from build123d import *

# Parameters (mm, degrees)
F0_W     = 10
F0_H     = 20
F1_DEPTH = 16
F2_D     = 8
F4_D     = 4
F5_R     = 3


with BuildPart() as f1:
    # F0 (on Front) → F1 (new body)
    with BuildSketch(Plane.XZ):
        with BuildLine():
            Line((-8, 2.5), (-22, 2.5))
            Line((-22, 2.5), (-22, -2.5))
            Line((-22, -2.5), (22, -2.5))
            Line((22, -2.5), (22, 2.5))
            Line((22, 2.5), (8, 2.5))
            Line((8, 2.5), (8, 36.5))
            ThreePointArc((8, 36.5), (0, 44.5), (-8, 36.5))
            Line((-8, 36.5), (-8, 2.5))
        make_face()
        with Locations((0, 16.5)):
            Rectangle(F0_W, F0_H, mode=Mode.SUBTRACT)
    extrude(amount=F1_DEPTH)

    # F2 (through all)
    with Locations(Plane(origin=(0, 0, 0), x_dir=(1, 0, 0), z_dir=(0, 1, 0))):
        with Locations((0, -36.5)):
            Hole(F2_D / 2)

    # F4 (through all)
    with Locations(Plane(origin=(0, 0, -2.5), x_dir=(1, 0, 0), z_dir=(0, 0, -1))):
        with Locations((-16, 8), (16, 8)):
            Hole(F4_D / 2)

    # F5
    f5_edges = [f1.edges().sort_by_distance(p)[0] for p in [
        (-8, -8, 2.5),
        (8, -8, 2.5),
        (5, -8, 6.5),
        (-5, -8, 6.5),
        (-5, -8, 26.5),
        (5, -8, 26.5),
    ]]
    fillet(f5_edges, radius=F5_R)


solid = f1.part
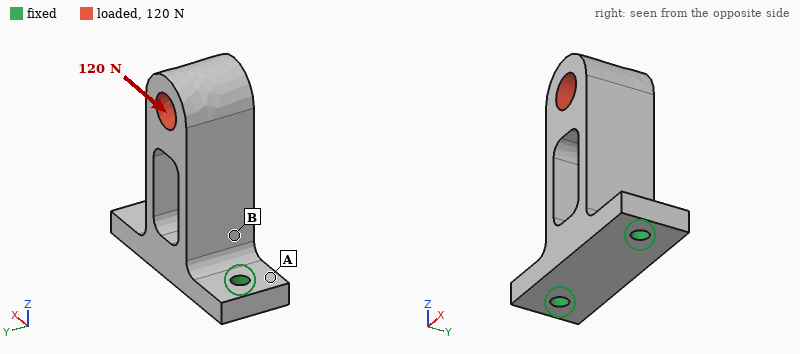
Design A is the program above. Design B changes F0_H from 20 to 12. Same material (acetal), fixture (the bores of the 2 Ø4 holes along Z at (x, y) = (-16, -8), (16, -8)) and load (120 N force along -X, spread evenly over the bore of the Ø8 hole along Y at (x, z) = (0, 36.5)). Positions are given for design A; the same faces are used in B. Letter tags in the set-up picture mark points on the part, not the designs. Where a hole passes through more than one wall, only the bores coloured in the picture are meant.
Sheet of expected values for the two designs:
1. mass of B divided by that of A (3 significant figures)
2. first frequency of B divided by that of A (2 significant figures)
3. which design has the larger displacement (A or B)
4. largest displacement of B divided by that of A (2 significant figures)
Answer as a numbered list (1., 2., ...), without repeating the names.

1. 1.13
2. 0.97
3. A
4. 0.60
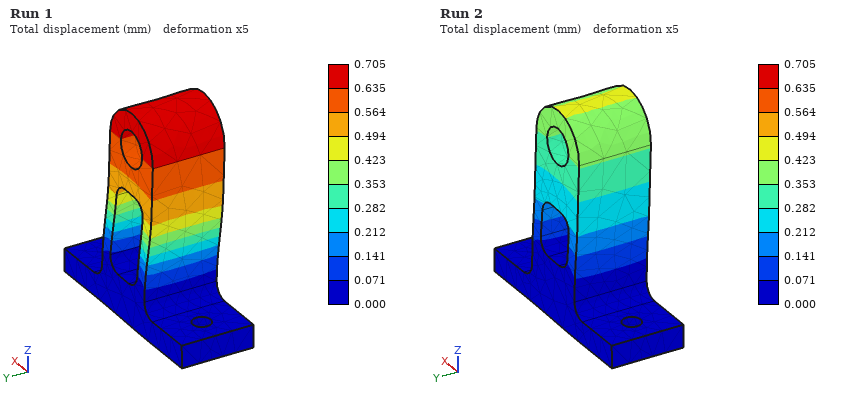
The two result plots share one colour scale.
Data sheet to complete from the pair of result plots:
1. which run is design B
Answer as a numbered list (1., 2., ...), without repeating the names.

1. Run 2
